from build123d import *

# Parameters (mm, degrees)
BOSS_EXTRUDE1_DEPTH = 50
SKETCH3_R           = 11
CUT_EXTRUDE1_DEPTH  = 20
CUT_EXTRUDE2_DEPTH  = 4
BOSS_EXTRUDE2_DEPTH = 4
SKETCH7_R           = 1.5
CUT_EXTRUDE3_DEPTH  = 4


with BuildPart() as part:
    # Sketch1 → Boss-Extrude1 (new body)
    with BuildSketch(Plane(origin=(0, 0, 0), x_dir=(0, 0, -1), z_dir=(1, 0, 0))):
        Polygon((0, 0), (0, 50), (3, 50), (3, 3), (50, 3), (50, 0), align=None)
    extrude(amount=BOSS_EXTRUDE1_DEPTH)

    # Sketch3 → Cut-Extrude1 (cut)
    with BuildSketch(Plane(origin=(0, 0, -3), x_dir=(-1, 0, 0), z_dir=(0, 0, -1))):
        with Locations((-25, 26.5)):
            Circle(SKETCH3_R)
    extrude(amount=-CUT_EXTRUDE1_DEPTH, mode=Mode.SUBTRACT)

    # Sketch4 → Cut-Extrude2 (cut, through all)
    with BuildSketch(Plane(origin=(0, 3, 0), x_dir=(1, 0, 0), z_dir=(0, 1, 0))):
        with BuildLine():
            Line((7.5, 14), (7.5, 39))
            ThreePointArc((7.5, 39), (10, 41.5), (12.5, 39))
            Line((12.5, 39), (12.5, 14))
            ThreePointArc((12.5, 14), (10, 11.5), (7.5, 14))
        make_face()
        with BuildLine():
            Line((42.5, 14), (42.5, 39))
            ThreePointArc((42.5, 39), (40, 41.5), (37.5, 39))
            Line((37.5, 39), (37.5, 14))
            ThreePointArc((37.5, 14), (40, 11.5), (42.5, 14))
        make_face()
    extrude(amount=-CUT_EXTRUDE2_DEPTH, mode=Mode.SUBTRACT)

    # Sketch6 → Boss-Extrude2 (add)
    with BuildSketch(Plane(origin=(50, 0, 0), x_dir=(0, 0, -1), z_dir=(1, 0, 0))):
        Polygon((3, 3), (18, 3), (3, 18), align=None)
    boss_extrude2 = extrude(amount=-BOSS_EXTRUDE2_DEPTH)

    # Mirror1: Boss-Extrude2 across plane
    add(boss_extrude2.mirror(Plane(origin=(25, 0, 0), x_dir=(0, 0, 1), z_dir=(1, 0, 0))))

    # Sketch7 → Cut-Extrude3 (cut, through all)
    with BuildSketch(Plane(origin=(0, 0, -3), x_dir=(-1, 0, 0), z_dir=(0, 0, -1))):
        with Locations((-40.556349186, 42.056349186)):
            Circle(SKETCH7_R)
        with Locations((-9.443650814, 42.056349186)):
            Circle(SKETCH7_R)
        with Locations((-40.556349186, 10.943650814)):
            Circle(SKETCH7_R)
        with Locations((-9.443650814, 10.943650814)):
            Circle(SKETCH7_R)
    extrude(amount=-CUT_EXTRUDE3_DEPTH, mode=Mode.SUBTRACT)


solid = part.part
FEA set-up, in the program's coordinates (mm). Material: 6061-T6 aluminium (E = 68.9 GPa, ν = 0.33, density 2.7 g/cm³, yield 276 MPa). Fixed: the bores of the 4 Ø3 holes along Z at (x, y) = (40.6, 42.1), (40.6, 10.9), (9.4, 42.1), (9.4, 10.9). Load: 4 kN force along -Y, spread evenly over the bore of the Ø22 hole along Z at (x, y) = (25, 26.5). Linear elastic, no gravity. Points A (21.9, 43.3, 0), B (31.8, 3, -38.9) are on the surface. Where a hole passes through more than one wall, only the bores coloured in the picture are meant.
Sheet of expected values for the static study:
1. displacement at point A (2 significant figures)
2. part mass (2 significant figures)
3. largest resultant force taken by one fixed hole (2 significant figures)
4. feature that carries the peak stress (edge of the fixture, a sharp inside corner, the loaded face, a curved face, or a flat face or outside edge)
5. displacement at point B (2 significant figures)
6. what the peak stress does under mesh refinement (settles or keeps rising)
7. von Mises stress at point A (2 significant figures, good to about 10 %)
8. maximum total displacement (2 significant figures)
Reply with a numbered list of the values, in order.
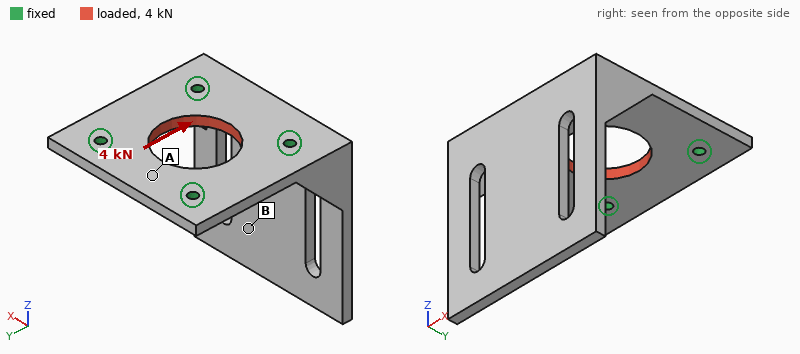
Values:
1. 8.8 µm
2. 36 g
3. 1.0 kN
4. edge of the fixture
5. 4.8 µm
6. keeps rising
7. 16 MPa
8. 11 µm
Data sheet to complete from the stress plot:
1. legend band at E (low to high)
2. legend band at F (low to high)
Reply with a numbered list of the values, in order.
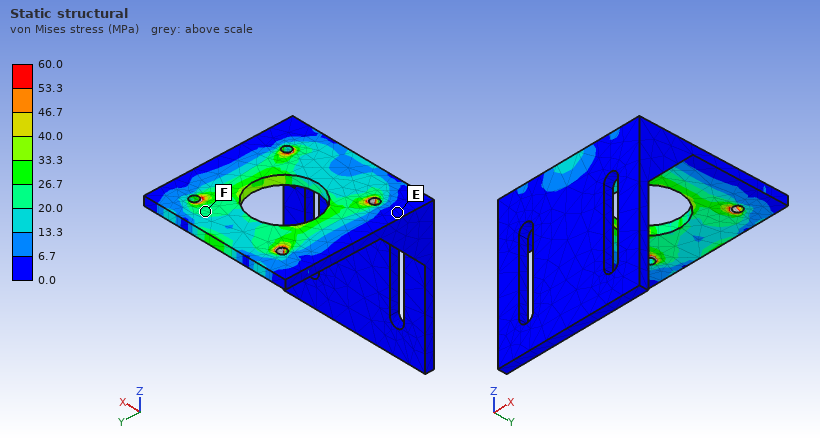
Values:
1. 0.0 to 6.7 MPa
2. 20.0 to 26.7 MPa
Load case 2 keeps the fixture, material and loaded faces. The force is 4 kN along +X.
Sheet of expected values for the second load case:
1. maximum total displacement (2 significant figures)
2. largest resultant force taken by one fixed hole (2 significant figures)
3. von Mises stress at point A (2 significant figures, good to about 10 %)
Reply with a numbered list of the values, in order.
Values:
1. 9.4 µm
2. 1.0 kN
3. 16 MPa
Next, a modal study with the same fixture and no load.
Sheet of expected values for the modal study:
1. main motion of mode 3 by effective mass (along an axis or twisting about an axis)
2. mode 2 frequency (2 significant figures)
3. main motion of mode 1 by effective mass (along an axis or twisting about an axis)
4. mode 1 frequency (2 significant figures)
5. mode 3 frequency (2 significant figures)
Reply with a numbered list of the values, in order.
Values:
1. along X
2. 2600 Hz
3. along Y
4. 1100 Hz
5. 4000 Hz
